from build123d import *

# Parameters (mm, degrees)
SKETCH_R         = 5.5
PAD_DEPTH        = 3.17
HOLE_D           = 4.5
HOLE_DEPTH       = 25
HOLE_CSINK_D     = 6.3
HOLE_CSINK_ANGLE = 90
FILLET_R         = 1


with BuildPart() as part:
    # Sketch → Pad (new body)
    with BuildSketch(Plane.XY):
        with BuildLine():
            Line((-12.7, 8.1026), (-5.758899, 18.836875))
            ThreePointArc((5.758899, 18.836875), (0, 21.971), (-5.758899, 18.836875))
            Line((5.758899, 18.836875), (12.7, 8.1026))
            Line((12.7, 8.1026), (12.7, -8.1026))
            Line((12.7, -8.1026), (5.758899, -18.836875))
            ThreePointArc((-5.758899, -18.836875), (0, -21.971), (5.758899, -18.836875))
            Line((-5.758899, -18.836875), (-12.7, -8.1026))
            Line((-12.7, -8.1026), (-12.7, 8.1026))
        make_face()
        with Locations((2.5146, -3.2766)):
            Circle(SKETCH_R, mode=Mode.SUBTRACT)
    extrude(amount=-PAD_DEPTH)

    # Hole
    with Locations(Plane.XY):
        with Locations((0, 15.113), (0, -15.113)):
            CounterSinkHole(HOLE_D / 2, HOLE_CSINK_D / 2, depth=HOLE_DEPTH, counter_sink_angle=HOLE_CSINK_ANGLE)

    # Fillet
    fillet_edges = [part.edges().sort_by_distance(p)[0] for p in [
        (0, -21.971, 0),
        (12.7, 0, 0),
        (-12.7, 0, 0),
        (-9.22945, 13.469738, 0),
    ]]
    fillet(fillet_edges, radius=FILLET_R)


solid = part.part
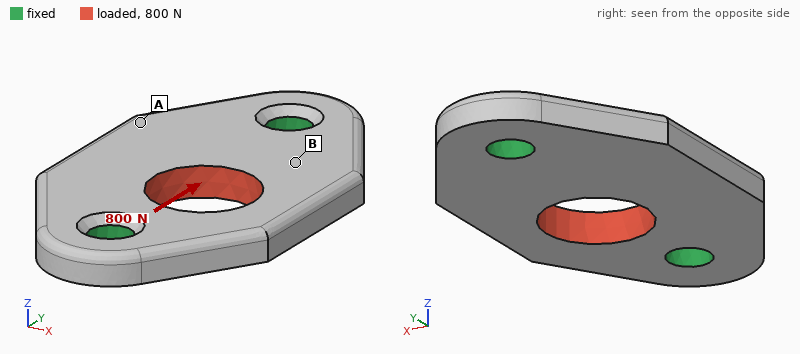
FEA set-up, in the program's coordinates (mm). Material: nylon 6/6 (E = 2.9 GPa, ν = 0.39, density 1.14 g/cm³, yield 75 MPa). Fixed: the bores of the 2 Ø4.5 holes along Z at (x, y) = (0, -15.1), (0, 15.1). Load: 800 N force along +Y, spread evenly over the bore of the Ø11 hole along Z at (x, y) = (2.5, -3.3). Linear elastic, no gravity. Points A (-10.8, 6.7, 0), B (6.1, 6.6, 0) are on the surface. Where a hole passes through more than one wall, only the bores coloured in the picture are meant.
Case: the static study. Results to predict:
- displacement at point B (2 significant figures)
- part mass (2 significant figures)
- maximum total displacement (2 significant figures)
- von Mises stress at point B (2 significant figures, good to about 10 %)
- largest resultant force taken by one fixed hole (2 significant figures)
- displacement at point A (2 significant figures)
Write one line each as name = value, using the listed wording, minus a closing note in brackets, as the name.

displacement at point B = 49 µm
part mass = 2.6 g
maximum total displacement = 81 µm
von Mises stress at point B = 8.9 MPa
largest resultant force taken by one fixed hole = 410 N
displacement at point A = 17 µm
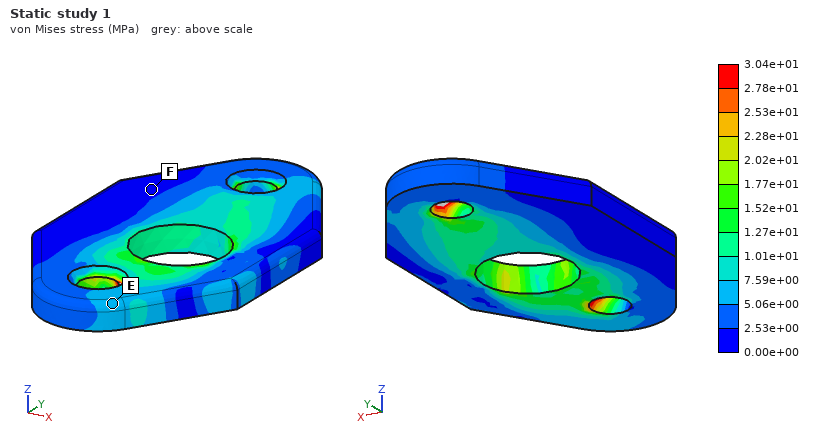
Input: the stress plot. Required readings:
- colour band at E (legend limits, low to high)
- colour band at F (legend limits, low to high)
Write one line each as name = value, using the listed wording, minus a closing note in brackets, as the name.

colour band at E = 5.06e+00 to 7.59e+00 MPa
colour band at F = 0.00e+00 to 2.53e+00 MPa
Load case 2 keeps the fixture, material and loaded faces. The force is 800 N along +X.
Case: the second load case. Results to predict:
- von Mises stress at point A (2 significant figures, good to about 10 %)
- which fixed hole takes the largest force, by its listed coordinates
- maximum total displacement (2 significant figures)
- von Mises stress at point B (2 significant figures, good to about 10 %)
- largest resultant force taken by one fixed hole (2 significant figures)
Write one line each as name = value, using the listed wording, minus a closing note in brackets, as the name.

von Mises stress at point A = 7.4 MPa
which fixed hole takes the largest force, by its listed coordinates = (0, -15.1)
maximum total displacement = 0.13 mm
von Mises stress at point B = 8.7 MPa
largest resultant force taken by one fixed hole = 480 N
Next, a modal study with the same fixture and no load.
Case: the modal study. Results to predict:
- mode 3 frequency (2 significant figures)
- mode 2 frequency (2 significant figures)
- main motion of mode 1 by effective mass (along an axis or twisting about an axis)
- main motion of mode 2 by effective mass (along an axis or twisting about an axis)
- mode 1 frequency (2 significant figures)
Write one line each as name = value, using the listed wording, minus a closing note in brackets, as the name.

mode 3 frequency = 8300 Hz
mode 2 frequency = 4000 Hz
main motion of mode 1 by effective mass = twisting about Y
main motion of mode 2 by effective mass = along Z
mode 1 frequency = 3500 Hz
